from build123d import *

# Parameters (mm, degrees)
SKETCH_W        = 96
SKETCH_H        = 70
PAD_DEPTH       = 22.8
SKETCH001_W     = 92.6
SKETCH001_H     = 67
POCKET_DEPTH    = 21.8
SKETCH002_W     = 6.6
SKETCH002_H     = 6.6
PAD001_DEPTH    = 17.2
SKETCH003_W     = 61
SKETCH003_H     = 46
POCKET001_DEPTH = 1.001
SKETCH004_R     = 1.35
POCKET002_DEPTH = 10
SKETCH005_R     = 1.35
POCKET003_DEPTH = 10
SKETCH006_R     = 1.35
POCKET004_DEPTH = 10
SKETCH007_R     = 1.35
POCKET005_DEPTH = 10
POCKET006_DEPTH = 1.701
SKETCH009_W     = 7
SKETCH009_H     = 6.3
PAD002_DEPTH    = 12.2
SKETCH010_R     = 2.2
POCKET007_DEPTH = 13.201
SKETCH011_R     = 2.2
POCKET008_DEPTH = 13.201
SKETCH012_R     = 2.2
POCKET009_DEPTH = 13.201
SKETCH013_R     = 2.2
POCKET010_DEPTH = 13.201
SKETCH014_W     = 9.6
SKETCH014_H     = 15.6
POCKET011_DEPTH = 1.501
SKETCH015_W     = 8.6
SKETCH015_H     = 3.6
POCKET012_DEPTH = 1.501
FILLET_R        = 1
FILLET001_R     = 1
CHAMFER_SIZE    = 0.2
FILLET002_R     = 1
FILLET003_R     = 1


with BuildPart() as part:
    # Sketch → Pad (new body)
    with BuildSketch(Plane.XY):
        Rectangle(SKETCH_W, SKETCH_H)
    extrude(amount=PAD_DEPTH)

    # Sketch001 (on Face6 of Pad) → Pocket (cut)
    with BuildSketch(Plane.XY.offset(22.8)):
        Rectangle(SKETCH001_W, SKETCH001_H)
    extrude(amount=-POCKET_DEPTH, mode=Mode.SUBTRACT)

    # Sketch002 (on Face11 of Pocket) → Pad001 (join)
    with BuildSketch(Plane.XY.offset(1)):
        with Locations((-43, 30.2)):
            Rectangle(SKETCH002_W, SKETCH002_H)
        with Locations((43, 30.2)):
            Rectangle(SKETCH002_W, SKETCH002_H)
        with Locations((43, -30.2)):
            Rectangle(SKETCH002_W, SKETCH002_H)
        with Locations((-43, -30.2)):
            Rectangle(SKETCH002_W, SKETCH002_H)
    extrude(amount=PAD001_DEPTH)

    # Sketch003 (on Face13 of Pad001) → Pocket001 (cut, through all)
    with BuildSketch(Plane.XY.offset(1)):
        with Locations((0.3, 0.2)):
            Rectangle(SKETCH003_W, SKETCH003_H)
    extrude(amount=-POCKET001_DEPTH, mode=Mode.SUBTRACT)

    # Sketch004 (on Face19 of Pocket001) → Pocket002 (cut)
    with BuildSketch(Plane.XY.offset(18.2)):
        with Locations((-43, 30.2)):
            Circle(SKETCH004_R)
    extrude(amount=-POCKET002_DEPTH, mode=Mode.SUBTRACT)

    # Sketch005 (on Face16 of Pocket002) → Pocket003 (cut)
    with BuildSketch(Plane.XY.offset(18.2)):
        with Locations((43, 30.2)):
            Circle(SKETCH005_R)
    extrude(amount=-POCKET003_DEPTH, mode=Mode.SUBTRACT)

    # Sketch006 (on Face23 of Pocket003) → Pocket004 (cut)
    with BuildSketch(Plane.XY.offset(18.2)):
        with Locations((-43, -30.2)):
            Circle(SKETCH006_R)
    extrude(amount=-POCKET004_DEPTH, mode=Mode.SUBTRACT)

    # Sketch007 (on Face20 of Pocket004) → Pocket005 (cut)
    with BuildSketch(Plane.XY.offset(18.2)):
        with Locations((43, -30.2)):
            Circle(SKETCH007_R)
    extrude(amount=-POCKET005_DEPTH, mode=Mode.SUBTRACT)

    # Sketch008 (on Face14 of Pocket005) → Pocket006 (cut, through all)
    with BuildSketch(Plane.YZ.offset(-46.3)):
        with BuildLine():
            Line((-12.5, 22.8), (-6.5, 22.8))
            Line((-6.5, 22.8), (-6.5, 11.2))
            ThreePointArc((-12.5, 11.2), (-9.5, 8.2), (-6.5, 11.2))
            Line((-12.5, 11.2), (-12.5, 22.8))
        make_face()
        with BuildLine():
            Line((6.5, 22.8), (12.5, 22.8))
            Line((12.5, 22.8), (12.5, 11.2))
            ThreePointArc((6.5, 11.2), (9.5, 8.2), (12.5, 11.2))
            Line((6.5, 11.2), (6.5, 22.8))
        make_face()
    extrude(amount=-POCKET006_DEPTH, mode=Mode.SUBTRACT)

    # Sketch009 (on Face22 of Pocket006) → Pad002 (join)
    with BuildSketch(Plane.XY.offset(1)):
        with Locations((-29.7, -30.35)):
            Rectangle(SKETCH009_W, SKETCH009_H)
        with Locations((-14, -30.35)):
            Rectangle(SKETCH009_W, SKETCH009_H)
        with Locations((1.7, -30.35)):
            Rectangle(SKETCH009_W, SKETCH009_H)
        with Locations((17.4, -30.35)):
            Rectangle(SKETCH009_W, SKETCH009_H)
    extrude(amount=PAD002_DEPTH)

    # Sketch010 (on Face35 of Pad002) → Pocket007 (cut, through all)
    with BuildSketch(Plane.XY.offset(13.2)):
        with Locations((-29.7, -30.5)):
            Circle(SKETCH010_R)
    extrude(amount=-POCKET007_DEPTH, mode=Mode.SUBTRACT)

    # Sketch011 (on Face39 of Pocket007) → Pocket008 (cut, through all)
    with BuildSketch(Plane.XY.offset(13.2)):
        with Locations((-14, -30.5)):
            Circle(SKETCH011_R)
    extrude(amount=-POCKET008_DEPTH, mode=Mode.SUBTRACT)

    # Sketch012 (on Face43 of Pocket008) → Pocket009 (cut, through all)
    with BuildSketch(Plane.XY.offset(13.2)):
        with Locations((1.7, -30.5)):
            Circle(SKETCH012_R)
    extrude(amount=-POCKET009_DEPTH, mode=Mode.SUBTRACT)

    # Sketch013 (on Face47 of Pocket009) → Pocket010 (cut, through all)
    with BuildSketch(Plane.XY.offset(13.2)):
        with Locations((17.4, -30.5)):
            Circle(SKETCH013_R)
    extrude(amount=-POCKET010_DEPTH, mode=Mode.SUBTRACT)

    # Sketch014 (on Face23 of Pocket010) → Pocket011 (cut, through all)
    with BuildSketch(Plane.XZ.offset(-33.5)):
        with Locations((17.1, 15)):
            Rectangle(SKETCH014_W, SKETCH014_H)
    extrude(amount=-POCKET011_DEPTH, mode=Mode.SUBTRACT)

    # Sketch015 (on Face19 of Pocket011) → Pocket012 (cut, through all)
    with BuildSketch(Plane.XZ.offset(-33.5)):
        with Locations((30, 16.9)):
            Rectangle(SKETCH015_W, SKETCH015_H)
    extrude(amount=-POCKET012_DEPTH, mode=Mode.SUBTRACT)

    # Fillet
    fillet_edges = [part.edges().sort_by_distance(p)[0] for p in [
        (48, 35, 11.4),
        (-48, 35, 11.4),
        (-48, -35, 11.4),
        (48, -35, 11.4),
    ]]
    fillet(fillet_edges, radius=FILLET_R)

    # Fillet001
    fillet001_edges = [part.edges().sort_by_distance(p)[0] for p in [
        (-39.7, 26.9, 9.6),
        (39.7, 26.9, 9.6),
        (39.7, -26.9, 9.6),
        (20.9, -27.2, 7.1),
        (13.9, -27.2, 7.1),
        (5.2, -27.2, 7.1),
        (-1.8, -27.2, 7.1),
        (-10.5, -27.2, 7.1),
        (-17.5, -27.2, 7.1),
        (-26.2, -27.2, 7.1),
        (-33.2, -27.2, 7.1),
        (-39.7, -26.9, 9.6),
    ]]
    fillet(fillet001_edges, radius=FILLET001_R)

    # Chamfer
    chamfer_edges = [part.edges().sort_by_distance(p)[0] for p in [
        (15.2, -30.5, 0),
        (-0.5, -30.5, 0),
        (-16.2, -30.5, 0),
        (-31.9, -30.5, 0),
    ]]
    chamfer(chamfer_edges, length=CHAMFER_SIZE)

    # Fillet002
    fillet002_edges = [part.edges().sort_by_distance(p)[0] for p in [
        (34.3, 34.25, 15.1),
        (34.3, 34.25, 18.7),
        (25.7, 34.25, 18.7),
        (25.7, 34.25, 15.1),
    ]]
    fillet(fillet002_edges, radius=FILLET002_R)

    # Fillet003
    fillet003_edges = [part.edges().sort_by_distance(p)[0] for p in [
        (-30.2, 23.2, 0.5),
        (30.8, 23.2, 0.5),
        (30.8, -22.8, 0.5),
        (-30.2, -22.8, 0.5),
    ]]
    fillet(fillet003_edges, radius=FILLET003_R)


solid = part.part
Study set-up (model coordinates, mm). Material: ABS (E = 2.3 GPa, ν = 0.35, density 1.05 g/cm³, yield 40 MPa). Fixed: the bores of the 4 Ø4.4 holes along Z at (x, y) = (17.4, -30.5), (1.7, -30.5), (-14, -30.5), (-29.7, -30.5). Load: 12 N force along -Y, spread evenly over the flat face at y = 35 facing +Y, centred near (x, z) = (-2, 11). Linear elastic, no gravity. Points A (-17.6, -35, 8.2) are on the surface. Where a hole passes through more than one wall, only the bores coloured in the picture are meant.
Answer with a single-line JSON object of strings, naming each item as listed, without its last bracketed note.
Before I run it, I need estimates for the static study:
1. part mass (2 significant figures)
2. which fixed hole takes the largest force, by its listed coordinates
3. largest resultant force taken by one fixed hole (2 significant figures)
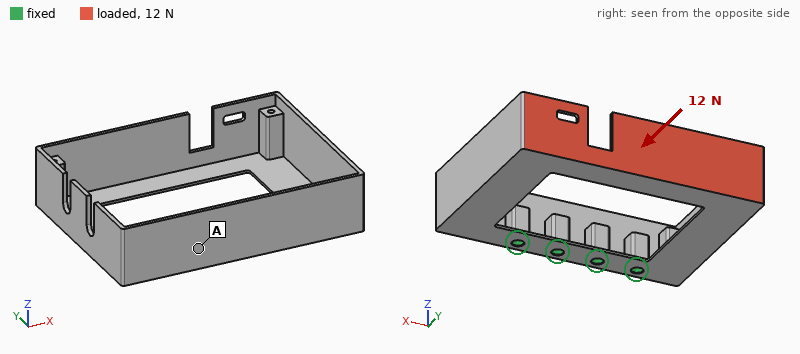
{"part mass": "20 g", "which fixed hole takes the largest force, by its listed coordinates": "(17.4, -30.5)", "largest resultant force taken by one fixed hole": "7.9 N"}
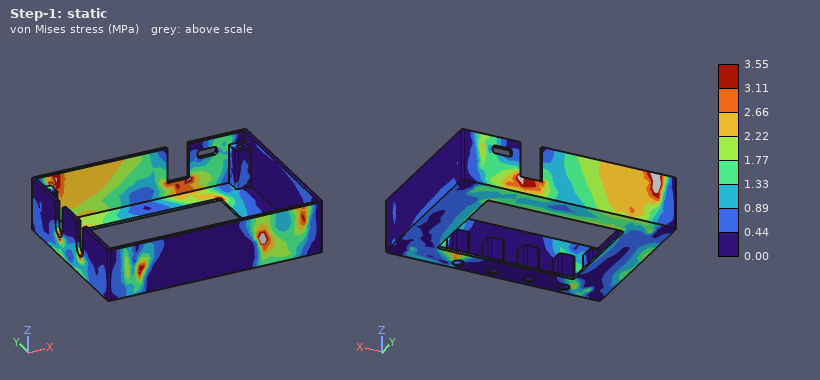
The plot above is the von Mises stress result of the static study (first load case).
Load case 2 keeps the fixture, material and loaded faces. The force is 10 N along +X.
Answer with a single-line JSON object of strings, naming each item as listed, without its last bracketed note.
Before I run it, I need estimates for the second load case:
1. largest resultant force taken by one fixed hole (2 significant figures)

{"largest resultant force taken by one fixed hole": "9.9 N"}
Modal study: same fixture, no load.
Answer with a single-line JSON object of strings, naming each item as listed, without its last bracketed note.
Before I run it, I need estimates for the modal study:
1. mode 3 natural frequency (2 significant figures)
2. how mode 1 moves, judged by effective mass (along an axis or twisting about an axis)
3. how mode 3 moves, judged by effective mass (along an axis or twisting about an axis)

{"mode 3 natural frequency": "320 Hz", "how mode 1 moves, judged by effective mass": "along Z", "how mode 3 moves, judged by effective mass": "along X"}
